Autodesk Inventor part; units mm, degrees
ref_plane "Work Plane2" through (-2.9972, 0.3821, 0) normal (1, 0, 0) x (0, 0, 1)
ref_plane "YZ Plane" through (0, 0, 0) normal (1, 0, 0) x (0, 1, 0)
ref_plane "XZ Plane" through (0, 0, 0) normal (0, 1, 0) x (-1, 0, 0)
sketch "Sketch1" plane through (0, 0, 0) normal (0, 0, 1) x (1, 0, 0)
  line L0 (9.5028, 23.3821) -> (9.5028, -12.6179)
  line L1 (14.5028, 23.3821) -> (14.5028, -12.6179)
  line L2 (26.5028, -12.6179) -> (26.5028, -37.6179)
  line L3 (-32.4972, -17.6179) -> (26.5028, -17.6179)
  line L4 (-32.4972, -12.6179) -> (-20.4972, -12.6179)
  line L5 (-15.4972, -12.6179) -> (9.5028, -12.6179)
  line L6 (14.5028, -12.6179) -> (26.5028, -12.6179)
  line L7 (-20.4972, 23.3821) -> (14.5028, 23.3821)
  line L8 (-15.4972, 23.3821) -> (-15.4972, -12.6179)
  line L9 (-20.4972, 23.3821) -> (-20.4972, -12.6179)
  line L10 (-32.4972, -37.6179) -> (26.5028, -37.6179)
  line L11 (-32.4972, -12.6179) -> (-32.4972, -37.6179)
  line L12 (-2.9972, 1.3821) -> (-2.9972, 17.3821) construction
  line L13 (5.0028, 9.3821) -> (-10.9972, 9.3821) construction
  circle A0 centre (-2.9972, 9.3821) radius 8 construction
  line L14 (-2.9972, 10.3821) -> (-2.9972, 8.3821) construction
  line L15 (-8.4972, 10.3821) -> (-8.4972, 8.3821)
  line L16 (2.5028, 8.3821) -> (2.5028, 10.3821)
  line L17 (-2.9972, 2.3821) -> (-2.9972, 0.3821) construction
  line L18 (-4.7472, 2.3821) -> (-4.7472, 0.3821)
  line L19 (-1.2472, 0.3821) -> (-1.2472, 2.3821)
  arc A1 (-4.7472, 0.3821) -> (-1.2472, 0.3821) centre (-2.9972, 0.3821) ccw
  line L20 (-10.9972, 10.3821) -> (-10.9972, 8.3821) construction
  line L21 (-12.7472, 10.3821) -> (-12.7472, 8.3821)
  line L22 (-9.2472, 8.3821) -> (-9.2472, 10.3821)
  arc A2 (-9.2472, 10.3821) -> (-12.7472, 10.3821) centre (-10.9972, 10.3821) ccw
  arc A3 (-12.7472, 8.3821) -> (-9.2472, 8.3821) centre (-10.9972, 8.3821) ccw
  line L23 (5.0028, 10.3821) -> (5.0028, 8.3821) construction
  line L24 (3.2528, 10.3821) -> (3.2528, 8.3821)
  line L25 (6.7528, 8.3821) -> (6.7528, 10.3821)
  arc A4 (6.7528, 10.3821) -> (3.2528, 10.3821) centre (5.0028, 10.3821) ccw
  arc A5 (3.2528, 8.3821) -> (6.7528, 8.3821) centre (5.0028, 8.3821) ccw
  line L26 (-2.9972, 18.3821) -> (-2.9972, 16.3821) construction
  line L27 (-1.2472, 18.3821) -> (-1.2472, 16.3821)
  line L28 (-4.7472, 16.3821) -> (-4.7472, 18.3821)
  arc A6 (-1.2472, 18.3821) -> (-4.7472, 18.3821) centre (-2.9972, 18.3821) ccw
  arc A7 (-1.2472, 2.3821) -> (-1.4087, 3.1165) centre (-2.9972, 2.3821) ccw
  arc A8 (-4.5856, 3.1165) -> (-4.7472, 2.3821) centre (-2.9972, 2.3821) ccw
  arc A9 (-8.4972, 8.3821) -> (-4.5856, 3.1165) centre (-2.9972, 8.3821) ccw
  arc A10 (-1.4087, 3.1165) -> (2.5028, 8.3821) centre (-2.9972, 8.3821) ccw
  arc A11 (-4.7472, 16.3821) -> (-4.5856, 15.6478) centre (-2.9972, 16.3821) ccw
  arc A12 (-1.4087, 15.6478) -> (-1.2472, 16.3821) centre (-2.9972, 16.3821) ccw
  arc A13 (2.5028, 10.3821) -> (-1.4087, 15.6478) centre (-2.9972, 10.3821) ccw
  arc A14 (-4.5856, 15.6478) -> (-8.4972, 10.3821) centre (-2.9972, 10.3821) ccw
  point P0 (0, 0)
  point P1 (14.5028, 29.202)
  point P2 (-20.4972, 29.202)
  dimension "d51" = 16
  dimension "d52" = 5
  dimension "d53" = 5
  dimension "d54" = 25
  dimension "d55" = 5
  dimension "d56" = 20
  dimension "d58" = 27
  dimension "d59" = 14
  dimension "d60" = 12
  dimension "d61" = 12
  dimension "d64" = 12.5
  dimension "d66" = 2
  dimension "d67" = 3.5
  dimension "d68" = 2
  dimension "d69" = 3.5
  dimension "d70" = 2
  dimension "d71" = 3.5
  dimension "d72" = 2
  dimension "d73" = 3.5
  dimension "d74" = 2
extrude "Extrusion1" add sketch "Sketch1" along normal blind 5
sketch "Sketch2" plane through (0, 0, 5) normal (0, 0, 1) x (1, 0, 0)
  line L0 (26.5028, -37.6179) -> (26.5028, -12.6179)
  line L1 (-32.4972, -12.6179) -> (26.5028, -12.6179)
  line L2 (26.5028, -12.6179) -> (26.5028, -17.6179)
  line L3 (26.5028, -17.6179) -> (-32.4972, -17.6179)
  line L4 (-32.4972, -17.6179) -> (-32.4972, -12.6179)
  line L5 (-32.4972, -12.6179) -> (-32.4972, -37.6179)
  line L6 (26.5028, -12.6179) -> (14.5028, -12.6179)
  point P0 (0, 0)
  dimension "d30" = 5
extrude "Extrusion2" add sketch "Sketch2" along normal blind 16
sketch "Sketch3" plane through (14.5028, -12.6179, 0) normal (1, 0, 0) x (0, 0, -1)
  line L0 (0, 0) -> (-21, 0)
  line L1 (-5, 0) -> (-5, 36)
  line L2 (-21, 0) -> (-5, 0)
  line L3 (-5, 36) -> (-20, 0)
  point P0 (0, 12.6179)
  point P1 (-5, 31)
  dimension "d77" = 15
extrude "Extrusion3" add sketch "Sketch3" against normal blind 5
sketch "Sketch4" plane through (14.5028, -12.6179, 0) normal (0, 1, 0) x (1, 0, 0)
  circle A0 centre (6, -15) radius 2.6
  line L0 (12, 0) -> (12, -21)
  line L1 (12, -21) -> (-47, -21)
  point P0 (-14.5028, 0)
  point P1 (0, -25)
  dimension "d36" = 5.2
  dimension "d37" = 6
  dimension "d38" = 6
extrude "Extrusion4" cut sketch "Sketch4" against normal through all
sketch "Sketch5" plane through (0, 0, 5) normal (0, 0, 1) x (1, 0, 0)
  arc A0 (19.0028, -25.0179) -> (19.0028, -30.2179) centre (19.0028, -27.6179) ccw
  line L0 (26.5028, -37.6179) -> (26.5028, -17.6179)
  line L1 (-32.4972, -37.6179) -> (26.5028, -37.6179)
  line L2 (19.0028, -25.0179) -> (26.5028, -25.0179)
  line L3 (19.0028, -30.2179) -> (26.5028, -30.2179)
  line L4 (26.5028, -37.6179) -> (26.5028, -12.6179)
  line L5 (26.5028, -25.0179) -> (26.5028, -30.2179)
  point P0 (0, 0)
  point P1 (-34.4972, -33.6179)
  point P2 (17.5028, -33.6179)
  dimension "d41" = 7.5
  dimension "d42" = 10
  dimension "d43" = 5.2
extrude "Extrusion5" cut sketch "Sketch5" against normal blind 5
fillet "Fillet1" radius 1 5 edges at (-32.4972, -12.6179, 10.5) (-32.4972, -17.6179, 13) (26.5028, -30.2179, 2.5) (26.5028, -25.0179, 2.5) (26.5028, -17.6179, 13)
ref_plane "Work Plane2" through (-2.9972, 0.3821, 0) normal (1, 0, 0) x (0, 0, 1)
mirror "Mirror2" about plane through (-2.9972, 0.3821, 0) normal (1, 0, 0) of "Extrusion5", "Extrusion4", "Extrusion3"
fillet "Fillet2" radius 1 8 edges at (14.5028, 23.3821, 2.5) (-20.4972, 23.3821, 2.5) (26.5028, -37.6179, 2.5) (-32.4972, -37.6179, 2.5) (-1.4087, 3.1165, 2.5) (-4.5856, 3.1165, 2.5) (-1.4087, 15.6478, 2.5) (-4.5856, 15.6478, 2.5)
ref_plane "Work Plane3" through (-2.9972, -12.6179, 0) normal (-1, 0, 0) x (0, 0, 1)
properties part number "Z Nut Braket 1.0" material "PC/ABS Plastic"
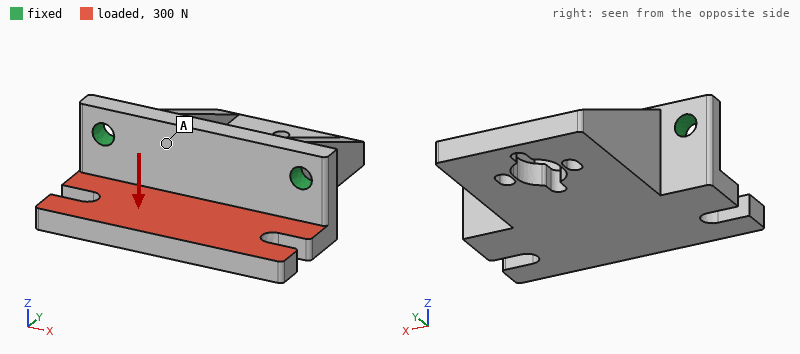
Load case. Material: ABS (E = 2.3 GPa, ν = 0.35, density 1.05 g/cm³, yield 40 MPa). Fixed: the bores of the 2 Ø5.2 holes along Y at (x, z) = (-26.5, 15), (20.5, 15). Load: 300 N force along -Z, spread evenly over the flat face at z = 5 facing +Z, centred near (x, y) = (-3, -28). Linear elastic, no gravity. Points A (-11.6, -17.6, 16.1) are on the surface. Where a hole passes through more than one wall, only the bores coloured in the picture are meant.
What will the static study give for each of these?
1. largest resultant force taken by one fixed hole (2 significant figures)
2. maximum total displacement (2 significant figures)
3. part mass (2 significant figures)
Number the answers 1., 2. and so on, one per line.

1. 170 N
2. 1.0 mm
3. 20 g
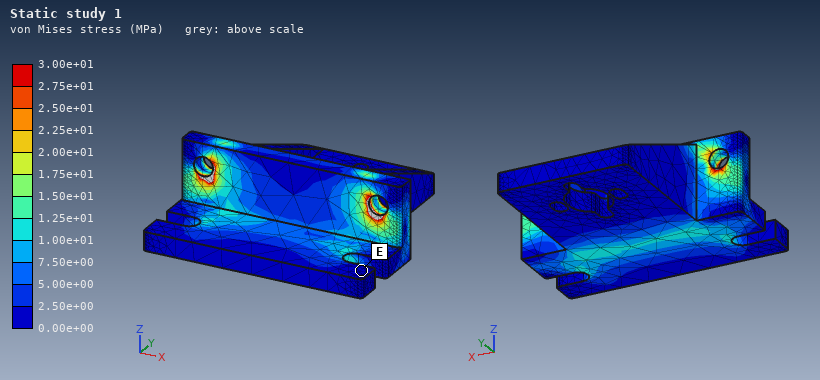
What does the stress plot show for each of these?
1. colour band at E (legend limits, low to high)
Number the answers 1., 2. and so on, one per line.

1. 0.00e+00 to 2.50e+00 MPa
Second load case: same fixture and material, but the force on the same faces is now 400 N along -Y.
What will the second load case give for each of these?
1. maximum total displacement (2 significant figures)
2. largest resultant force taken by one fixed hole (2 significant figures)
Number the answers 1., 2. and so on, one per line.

1. 0.59 mm
2. 200 N
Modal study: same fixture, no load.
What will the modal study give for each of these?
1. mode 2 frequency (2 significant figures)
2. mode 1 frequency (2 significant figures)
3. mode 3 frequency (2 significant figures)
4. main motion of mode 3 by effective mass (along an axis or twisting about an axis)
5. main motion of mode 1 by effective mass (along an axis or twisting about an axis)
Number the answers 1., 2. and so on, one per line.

1. 1700 Hz
2. 880 Hz
3. 2100 Hz
4. along Z
5. along Y
